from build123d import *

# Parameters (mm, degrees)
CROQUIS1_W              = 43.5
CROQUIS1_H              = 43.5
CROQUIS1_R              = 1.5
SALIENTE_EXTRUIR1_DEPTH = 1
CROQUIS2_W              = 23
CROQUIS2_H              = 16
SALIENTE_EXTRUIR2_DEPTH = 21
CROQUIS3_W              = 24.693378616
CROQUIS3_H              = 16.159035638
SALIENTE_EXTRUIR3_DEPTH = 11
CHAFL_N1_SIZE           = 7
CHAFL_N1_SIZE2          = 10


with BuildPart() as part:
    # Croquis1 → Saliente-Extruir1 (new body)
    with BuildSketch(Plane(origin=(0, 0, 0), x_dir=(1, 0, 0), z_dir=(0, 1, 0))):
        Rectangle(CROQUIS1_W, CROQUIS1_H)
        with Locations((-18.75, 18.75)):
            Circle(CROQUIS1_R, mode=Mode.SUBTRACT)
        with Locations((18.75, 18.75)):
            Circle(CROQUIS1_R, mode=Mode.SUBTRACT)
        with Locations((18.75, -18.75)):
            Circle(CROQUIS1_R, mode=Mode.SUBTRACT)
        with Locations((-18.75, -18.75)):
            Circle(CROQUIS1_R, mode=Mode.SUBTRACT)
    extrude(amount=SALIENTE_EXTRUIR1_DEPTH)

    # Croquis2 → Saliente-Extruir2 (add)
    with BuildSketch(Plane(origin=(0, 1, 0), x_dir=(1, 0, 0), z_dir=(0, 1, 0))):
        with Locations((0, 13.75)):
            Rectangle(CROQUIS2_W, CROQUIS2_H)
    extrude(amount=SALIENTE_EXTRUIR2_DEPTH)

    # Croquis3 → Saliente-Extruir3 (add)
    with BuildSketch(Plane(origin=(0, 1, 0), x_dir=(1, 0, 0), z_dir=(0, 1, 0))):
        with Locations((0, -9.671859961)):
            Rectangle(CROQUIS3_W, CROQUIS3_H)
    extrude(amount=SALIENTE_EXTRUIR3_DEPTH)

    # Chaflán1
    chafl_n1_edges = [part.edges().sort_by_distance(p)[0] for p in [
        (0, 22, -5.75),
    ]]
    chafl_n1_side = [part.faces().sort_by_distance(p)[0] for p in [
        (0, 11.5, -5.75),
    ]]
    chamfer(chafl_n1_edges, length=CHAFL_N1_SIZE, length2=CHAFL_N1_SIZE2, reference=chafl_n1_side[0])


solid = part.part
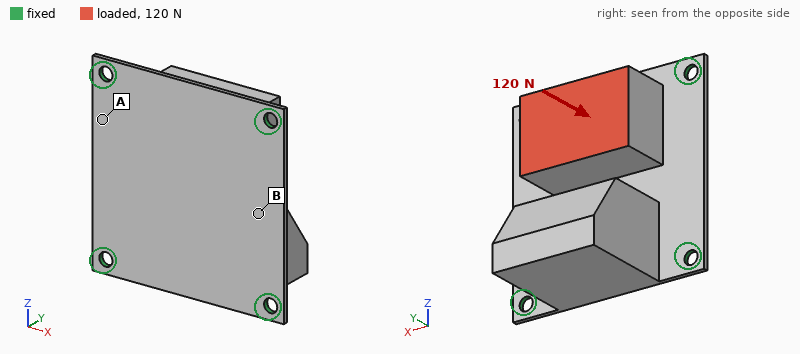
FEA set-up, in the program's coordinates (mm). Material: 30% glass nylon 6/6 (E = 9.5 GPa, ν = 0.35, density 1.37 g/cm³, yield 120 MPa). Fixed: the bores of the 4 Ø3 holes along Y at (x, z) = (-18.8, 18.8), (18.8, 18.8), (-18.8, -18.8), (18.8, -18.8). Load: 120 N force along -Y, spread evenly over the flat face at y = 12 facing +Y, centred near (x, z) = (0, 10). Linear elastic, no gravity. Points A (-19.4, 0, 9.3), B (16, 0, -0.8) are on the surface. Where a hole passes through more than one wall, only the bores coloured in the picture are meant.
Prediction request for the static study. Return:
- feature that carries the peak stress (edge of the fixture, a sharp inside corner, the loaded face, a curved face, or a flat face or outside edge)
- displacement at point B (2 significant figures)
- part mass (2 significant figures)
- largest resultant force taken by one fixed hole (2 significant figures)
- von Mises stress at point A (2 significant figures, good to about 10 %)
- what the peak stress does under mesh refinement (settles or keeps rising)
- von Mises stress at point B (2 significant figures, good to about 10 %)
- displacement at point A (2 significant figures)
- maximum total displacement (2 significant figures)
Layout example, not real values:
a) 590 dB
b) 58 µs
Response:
a) edge of the fixture
b) 0.45 mm
c) 18 g
d) 51 N
e) 9.7 MPa
f) keeps rising
g) 26 MPa
h) 0.22 mm
i) 0.66 mm
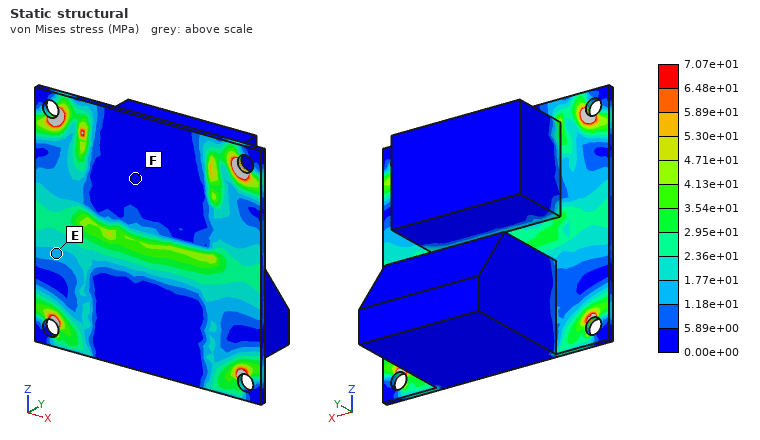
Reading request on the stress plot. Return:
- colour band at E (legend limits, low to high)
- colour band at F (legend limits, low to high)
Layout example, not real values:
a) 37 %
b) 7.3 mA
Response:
a) 1.18e+01 to 1.77e+01 MPa
b) 0.00e+00 to 5.89e+00 MPa
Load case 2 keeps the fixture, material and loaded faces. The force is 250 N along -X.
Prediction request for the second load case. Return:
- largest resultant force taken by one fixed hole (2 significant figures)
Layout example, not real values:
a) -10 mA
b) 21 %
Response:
a) 120 N
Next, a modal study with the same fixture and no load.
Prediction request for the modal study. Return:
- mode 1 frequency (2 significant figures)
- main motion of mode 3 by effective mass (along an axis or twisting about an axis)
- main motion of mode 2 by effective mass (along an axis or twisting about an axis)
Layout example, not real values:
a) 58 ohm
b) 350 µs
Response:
a) 520 Hz
b) along X
c) along Y
